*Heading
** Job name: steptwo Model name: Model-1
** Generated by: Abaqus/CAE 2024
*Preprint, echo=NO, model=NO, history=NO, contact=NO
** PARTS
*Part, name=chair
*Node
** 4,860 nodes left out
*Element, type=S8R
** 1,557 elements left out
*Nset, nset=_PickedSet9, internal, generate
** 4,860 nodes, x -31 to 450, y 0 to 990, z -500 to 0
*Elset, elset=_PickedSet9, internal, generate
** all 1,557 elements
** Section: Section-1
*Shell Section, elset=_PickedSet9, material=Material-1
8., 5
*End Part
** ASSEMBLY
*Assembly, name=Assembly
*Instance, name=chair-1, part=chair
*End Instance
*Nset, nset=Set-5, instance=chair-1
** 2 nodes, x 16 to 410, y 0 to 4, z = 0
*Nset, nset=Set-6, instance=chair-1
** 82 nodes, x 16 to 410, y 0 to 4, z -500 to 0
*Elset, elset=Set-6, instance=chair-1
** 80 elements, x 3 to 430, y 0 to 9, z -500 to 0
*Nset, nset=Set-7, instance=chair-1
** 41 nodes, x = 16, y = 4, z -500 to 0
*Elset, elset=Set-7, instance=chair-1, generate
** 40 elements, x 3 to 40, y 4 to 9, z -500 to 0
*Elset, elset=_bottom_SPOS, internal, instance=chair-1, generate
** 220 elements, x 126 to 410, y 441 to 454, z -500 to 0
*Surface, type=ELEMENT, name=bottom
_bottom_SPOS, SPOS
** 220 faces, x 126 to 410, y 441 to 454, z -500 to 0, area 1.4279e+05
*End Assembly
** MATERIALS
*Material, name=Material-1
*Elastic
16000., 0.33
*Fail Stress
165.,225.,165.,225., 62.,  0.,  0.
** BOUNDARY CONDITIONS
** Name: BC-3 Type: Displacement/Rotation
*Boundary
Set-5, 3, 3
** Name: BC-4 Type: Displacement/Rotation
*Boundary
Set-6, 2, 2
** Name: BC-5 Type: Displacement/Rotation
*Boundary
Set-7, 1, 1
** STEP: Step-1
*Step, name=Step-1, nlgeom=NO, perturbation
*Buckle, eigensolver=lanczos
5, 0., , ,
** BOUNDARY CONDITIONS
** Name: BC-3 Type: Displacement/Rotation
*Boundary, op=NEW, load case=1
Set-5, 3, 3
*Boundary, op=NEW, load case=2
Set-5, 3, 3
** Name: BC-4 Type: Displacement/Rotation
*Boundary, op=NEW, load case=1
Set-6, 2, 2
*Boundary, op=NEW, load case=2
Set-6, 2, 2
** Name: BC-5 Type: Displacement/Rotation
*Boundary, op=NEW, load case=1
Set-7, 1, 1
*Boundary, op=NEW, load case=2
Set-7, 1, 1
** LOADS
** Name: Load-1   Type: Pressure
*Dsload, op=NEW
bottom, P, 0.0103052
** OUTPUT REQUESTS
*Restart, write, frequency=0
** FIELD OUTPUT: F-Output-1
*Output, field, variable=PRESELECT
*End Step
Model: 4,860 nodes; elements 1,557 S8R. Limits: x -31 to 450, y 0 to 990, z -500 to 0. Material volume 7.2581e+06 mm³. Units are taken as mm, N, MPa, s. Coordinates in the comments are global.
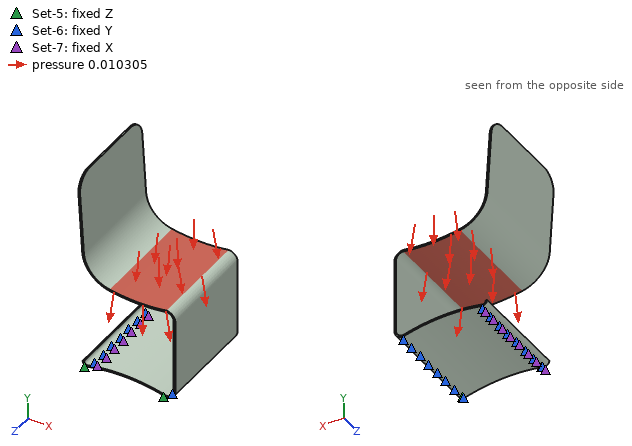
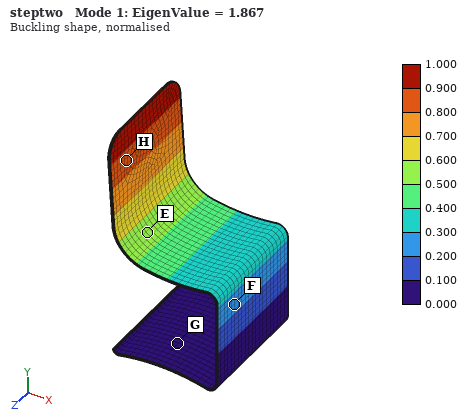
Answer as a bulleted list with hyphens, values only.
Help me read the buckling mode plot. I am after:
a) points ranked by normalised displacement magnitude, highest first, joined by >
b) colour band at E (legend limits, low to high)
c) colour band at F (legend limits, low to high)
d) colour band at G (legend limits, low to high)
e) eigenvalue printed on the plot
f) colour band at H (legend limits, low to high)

- H > E > F > G
- 0.500 to 0.600
- 0.200 to 0.300
- 0.000 to 0.100
- 1.867
- 0.800 to 0.900
